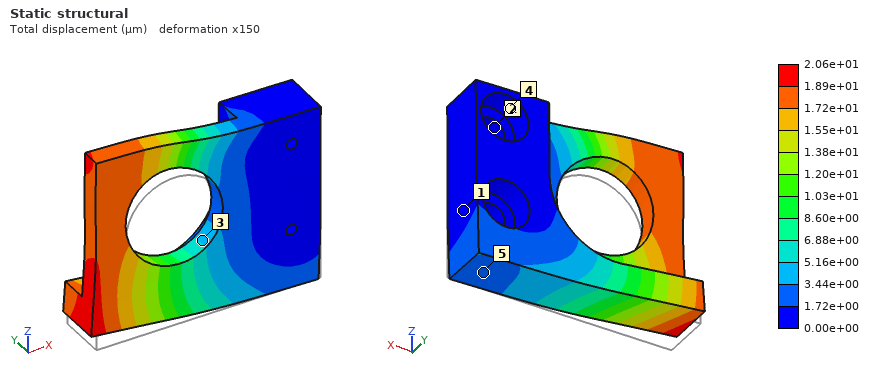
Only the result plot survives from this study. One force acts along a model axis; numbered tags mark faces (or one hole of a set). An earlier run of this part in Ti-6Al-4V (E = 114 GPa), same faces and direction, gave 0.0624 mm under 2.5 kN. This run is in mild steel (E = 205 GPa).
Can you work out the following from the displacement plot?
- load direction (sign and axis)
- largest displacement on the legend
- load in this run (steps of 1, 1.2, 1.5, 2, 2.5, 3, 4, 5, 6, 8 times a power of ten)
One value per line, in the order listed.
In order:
+Z
2.06e+01 µm
1.5 kN
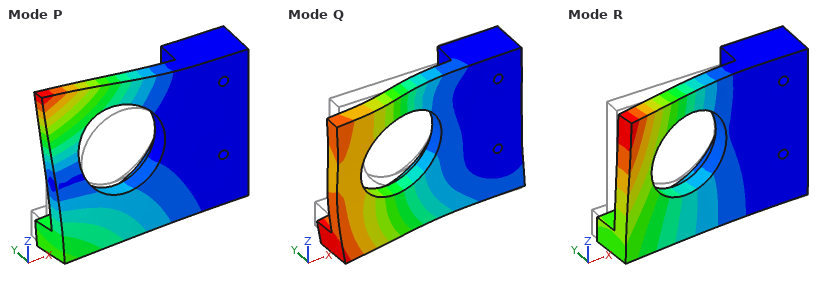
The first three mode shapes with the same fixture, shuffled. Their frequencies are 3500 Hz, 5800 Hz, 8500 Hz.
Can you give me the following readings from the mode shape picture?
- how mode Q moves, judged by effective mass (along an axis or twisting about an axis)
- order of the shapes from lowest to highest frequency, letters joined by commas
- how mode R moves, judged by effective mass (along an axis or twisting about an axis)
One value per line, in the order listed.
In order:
along Z
R, P, Q
along Y
